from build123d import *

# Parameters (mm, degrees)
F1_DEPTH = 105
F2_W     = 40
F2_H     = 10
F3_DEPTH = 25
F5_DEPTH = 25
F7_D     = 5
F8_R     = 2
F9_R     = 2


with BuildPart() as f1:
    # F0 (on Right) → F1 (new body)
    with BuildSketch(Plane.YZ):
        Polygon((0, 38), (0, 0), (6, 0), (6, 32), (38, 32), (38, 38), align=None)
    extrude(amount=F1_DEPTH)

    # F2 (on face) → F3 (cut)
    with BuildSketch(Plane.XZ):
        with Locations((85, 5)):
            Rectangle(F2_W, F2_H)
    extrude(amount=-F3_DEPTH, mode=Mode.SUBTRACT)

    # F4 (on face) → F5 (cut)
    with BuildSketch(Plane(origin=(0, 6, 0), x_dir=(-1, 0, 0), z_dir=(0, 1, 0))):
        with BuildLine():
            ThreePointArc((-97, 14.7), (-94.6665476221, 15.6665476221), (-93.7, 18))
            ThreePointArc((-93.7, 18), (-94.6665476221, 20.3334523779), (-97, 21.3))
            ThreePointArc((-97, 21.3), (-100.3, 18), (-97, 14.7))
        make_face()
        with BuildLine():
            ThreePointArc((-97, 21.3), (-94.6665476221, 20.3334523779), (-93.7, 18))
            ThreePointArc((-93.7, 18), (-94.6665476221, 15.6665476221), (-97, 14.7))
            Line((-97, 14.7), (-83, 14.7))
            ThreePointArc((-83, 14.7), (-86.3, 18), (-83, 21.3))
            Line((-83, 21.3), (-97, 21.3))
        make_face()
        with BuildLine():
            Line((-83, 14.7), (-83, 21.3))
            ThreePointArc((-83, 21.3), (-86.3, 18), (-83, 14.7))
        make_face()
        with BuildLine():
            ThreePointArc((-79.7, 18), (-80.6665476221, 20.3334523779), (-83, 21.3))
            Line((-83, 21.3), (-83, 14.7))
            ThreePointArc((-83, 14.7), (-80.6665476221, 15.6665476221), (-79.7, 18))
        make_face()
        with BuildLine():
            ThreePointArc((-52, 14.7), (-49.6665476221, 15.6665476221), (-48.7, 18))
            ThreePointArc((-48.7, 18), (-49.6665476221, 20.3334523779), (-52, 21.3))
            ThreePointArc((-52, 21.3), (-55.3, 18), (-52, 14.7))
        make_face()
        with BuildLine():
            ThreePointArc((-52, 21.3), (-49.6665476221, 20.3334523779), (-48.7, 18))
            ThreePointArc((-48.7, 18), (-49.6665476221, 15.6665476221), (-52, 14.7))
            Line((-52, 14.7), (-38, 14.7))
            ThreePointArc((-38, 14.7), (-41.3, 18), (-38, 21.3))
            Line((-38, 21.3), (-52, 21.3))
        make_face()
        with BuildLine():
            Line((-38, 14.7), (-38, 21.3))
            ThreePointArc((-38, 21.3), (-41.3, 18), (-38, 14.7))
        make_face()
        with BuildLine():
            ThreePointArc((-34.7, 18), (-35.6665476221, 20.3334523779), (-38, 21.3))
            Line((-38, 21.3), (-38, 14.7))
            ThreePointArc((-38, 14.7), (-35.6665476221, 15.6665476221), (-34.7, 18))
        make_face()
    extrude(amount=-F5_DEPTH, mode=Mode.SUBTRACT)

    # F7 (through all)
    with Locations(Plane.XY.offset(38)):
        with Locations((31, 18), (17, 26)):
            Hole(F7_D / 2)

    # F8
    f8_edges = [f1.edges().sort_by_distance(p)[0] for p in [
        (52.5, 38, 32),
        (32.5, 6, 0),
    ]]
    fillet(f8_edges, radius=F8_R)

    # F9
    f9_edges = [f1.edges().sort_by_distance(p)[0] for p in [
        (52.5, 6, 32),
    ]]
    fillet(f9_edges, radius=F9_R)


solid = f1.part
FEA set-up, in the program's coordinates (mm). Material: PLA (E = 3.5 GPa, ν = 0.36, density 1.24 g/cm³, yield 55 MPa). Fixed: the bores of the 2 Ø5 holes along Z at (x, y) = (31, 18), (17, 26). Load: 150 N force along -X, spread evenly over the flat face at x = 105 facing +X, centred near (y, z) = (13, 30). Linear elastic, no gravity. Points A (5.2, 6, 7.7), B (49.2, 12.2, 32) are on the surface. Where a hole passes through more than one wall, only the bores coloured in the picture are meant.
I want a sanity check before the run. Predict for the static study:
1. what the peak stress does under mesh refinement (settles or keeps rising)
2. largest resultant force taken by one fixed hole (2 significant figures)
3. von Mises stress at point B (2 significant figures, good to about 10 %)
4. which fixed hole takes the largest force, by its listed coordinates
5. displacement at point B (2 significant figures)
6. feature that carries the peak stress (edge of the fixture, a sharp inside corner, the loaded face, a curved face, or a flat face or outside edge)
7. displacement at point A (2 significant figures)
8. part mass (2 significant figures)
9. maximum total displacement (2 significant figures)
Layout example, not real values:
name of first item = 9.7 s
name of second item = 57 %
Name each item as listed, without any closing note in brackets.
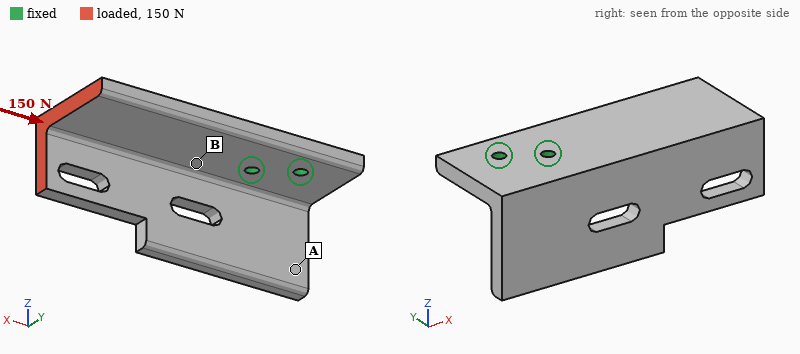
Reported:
what the peak stress does under mesh refinement = keeps rising
largest resultant force taken by one fixed hole = 140 N
von Mises stress at point B = 0.75 MPa
which fixed hole takes the largest force, by its listed coordinates = (31, 18)
displacement at point B = 0.026 mm
feature that carries the peak stress = edge of the fixture
displacement at point A = 0.067 mm
part mass = 49 g
maximum total displacement = 0.14 mm
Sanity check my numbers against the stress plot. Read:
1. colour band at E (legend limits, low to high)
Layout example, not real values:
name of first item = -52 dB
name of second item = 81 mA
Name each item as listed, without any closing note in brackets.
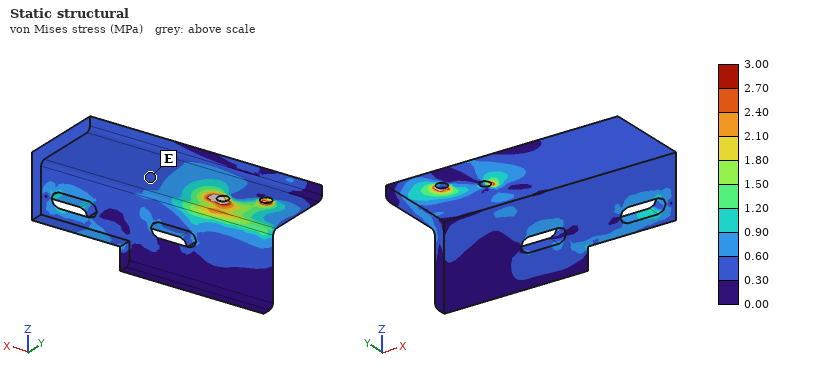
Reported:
colour band at E = 0.30 to 0.60 MPa
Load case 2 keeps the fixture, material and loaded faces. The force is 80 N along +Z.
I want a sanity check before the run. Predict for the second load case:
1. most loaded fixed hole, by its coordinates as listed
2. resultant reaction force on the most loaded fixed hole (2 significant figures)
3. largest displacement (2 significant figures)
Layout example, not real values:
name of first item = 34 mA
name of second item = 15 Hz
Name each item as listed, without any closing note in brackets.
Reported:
most loaded fixed hole, by its coordinates as listed = (31, 18)
resultant reaction force on the most loaded fixed hole = 270 N
largest displacement = 1.2 mm
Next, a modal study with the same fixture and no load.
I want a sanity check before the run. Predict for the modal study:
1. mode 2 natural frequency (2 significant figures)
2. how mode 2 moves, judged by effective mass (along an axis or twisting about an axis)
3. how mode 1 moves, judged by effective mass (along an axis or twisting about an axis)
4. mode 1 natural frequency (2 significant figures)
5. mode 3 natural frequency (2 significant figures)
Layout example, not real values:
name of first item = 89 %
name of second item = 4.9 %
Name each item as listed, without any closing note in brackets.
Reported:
mode 2 natural frequency = 620 Hz
how mode 2 moves, judged by effective mass = along Y
how mode 1 moves, judged by effective mass = along Z
mode 1 natural frequency = 410 Hz
mode 3 natural frequency = 940 Hz
